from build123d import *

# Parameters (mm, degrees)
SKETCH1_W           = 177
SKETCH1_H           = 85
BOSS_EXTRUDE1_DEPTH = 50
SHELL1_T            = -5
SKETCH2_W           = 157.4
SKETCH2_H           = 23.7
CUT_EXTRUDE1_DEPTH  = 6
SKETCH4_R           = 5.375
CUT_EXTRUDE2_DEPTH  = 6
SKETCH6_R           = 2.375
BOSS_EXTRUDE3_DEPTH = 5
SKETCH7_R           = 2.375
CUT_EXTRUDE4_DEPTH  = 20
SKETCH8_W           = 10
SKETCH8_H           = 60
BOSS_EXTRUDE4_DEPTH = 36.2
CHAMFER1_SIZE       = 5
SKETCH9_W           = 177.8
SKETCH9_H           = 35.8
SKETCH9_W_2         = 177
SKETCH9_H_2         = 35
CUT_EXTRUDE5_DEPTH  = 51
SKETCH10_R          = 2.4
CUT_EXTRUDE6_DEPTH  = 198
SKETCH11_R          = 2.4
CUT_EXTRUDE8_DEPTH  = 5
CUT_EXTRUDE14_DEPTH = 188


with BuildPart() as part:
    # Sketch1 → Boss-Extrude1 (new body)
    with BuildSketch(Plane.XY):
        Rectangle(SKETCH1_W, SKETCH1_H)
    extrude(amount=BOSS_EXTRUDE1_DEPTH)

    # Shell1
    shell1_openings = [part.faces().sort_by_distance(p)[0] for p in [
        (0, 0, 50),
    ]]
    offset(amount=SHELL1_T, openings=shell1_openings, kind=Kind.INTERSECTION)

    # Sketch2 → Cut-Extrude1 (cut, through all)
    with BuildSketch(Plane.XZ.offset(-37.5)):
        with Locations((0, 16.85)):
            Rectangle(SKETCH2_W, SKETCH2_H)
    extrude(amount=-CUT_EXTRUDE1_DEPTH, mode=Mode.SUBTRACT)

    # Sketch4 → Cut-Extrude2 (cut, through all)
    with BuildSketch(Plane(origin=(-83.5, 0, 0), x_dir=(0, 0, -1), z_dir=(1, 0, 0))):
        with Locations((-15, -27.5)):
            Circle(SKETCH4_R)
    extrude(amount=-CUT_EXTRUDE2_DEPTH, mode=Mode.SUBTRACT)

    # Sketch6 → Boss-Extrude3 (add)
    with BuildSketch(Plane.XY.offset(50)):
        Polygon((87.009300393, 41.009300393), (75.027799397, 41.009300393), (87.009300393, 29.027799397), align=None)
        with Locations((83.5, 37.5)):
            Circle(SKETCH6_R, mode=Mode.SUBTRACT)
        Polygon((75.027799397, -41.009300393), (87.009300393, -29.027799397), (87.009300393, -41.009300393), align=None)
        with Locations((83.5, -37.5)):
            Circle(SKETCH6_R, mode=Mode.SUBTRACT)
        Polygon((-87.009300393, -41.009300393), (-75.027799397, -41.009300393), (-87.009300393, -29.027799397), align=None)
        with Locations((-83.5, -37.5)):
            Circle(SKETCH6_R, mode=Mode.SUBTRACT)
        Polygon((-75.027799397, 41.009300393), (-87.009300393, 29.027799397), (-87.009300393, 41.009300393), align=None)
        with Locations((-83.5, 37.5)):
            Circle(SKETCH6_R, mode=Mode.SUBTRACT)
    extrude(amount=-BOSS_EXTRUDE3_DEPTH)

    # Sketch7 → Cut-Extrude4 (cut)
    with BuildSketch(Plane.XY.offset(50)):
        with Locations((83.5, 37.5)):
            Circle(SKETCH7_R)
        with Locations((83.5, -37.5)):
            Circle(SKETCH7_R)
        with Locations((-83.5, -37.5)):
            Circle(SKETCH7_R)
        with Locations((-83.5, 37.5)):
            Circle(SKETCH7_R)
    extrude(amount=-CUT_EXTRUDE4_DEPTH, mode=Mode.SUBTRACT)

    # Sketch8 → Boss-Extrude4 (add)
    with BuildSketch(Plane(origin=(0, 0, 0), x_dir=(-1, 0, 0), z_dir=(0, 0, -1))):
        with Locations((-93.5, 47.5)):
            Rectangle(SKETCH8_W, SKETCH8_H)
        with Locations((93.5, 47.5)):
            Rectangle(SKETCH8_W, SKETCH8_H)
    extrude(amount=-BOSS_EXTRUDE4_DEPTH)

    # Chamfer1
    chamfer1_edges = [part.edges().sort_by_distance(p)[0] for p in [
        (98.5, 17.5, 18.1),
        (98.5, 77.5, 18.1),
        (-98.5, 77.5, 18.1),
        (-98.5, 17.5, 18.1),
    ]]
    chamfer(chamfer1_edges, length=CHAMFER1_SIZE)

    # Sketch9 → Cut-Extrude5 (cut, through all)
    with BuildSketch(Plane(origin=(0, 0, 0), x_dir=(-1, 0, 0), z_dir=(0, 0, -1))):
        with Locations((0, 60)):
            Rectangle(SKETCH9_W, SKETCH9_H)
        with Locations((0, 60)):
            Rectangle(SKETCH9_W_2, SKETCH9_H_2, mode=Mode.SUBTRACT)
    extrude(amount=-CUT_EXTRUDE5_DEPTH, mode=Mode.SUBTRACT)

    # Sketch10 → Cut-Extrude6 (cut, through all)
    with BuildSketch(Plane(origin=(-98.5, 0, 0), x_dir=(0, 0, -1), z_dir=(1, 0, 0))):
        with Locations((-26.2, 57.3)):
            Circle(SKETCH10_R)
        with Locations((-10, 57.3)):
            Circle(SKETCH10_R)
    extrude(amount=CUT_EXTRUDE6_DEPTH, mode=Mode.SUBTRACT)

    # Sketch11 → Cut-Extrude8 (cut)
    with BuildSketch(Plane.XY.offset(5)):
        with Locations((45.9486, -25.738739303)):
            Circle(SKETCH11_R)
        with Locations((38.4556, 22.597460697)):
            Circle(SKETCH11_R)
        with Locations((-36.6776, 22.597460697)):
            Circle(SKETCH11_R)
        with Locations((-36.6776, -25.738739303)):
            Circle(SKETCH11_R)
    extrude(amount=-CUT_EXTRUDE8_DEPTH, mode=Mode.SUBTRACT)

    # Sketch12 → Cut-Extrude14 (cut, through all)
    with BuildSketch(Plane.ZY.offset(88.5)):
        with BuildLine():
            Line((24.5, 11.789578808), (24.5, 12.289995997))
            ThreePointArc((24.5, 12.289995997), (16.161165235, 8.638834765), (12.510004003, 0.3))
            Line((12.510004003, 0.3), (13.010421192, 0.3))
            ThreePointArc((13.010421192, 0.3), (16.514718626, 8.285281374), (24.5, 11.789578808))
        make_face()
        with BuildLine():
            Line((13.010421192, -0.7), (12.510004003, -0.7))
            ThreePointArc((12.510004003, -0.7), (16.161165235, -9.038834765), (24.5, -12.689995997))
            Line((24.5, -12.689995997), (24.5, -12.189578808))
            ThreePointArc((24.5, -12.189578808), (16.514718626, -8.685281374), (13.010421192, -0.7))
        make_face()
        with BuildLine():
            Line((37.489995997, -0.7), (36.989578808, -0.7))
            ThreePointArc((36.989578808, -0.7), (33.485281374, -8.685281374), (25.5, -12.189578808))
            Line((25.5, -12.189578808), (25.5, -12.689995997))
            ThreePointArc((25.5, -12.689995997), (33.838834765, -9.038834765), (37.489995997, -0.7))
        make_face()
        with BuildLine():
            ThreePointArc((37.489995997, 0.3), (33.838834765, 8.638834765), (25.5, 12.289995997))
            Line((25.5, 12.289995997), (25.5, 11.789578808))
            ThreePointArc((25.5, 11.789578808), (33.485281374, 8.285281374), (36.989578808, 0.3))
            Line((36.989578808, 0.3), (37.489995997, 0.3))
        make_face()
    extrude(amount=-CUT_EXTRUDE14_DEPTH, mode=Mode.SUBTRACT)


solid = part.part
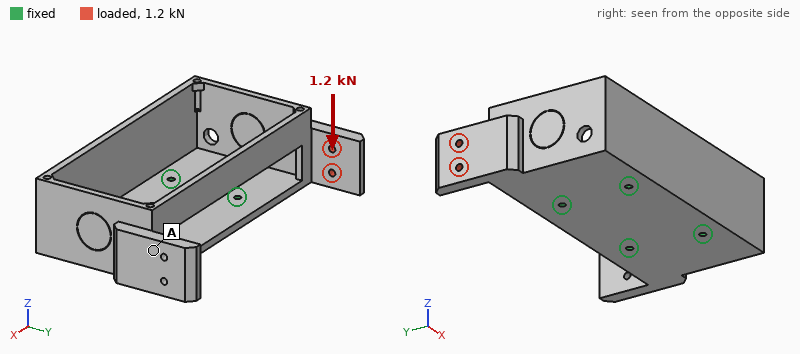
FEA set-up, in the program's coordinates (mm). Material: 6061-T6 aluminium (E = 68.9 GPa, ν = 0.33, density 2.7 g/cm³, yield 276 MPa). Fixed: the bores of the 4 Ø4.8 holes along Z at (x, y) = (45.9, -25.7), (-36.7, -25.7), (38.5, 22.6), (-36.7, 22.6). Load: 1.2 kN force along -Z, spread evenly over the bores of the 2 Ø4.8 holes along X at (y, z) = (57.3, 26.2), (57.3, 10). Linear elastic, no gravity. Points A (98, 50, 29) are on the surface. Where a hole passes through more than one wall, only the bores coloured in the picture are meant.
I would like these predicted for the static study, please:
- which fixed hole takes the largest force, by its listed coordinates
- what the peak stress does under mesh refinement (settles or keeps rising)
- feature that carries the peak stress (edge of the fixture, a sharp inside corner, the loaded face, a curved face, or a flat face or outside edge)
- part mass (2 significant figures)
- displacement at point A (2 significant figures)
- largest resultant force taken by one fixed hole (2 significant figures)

(-36.7, 22.6)
keeps rising
edge of the fixture
560 g
0.29 mm
1.9 kN
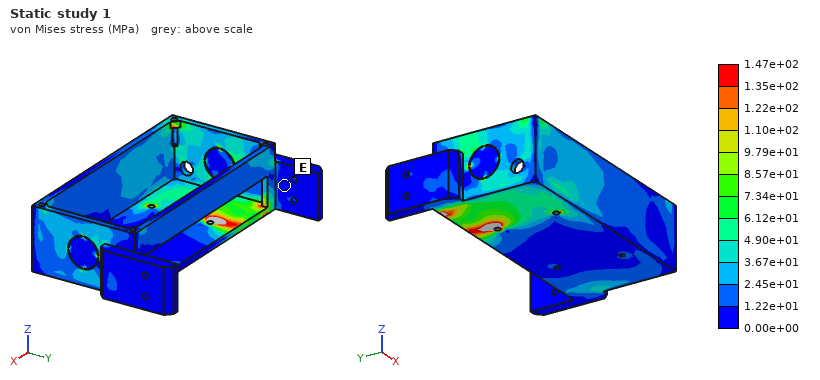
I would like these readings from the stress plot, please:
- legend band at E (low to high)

0.00e+00 to 1.22e+01 MPa
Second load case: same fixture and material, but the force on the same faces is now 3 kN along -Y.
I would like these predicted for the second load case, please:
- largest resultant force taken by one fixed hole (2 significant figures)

3.2 kN
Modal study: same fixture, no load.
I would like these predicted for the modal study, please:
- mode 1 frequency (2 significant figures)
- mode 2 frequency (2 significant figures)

560 Hz
630 Hz
